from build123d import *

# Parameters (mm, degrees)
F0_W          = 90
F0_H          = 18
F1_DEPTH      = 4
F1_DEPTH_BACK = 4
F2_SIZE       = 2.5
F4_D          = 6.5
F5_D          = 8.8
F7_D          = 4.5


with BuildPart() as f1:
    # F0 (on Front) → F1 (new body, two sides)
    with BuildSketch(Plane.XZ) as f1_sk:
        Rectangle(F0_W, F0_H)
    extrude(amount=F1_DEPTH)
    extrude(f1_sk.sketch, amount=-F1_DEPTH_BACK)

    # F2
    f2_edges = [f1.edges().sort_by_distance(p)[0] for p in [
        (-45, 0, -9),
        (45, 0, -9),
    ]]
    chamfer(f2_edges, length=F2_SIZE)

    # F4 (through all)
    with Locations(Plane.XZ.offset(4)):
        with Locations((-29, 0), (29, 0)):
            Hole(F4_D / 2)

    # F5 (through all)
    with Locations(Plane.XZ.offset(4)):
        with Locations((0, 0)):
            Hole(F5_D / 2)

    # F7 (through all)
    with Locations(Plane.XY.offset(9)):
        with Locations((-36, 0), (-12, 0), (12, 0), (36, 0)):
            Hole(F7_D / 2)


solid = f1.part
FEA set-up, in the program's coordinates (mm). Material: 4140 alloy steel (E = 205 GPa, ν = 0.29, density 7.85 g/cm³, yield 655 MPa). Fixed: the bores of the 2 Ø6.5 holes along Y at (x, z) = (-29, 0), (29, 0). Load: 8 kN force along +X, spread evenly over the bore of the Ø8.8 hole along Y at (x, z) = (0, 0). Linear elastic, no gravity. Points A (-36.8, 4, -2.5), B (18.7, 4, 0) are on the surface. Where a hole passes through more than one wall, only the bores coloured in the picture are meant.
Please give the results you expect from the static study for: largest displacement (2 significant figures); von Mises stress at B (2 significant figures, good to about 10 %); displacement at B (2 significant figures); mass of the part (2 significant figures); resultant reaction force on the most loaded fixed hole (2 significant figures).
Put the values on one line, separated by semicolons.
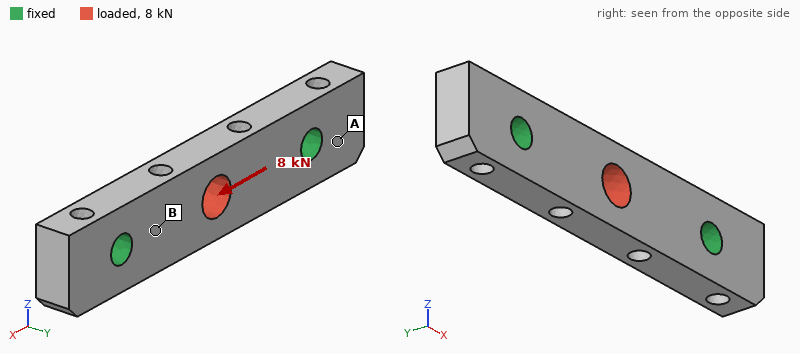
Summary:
5.3 µm; 41 MPa; 1.4 µm; 84 g; 4.0 kN
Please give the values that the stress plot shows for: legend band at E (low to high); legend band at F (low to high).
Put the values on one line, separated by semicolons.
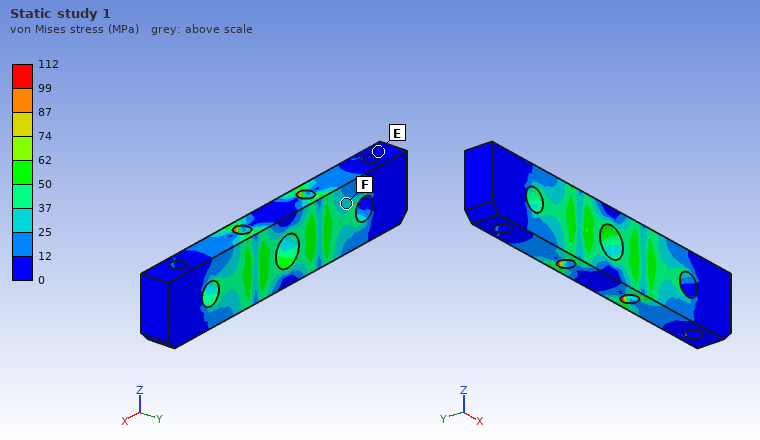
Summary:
0 to 12 MPa; 25 to 37 MPa
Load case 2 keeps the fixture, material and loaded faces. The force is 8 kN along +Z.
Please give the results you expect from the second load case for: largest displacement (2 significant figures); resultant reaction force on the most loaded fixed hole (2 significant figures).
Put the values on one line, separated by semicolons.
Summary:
28 µm; 4.0 kN
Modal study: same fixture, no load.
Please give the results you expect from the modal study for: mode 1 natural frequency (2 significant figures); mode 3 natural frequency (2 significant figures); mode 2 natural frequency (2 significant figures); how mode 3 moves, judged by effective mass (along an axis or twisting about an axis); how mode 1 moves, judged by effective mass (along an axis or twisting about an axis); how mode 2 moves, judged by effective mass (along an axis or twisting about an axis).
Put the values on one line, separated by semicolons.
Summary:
12 kHz; 20 kHz; 17 kHz; twisting about X; along Y; along Z
